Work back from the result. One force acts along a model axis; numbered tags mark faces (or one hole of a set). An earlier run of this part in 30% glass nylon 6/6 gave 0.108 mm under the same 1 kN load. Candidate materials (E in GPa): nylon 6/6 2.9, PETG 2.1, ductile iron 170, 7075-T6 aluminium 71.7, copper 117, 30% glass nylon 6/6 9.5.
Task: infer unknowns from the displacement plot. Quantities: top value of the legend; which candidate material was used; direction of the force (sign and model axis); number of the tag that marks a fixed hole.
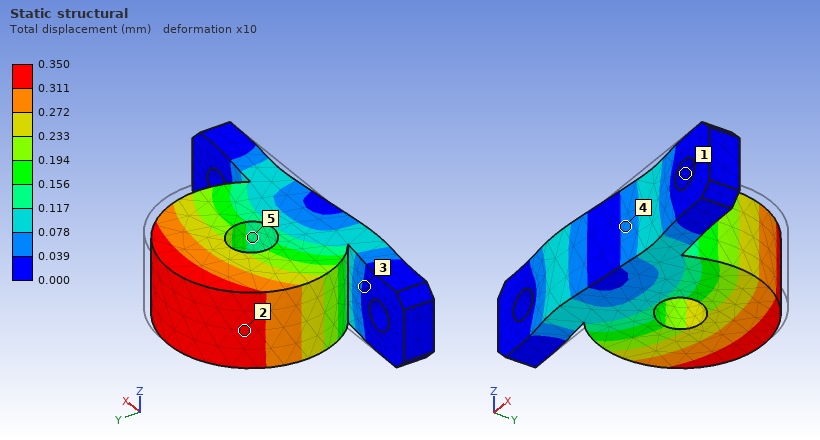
0.350 mm
nylon 6/6
-X
1
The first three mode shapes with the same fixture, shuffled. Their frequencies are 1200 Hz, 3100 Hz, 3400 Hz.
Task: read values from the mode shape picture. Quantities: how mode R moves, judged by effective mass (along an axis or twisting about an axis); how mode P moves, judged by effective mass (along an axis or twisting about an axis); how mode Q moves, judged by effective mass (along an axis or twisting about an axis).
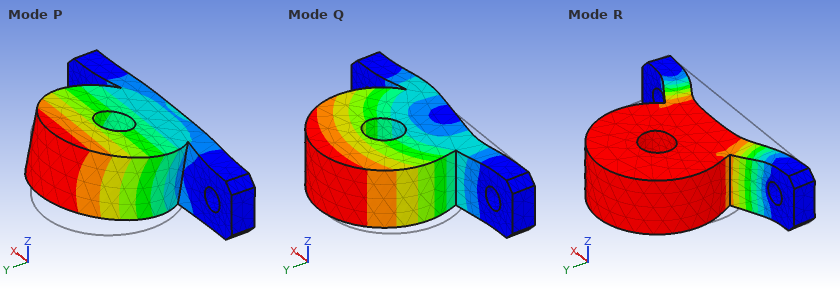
along Y
along Z
along X
